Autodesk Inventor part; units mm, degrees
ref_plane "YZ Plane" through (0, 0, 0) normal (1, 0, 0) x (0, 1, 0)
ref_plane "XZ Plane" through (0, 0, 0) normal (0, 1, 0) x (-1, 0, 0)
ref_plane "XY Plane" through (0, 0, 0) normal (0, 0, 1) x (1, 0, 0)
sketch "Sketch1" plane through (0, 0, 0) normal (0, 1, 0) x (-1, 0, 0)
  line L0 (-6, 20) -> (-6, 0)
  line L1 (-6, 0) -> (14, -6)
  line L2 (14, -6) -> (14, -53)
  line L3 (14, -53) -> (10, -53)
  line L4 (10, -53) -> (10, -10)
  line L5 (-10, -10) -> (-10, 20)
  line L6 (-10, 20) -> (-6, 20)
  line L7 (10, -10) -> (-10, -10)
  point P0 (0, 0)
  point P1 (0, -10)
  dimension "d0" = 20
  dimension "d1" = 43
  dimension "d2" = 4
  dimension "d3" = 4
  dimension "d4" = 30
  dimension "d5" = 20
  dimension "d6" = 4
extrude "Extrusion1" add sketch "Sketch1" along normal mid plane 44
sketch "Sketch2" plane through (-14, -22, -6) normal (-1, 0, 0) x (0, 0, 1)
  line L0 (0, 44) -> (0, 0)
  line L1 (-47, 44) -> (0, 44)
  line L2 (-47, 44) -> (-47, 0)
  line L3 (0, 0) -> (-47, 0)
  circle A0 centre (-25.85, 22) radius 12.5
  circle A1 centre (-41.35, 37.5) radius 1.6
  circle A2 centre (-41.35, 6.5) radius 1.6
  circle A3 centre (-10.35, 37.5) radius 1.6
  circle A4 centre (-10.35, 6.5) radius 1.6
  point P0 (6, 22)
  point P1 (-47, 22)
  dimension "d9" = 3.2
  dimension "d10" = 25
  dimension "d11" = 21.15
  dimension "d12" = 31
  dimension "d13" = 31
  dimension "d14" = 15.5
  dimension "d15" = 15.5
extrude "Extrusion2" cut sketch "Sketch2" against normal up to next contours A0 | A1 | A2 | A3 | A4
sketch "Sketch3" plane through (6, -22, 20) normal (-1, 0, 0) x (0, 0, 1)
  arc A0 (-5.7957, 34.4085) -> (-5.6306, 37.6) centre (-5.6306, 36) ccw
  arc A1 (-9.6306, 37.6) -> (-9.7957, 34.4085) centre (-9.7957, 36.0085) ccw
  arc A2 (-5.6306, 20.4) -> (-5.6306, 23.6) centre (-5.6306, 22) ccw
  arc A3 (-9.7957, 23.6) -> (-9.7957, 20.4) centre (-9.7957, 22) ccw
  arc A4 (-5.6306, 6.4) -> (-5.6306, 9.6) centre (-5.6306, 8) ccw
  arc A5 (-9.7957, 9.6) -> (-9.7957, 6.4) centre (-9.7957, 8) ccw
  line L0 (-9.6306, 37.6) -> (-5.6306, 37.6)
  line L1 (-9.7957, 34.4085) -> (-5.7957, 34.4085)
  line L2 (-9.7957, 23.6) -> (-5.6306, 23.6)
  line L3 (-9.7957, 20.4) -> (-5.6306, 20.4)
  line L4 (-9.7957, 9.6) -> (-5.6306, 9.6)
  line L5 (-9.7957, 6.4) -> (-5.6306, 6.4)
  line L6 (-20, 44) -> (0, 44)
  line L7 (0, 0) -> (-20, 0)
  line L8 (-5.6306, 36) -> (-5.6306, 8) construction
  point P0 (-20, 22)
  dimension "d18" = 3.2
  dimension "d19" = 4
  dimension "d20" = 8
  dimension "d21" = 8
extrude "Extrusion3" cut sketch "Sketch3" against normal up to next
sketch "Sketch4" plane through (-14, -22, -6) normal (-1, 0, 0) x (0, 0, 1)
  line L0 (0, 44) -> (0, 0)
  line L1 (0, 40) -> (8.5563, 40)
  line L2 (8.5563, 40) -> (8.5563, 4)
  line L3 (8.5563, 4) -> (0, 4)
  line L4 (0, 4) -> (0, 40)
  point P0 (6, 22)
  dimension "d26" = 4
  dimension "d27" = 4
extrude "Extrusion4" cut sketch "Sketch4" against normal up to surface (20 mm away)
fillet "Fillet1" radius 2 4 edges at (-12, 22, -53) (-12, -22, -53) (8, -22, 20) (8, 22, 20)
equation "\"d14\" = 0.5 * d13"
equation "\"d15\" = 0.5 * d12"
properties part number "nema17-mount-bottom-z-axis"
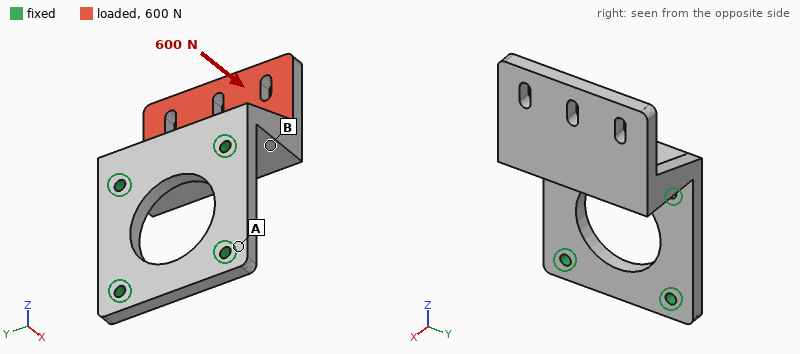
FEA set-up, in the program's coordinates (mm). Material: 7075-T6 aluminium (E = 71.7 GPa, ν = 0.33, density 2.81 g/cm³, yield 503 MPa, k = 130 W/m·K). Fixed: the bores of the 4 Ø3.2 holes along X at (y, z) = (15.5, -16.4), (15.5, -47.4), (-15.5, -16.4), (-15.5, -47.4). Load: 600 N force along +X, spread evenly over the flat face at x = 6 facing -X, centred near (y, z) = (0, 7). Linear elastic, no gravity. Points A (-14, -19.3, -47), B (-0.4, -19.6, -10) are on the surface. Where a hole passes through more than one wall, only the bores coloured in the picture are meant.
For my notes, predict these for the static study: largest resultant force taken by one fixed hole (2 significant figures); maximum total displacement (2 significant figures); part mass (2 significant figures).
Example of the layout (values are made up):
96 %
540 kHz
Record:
350 N
0.49 mm
41 g
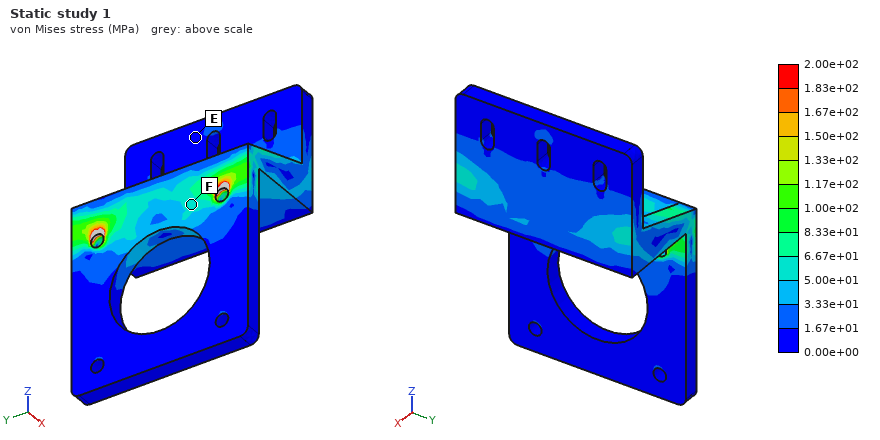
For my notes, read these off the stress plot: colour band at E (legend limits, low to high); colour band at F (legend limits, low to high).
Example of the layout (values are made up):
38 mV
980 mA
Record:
0.00e+00 to 1.67e+01 MPa
5.00e+01 to 6.67e+01 MPa
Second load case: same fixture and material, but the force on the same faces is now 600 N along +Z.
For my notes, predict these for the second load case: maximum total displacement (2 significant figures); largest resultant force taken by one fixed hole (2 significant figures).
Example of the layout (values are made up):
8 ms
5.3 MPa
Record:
0.33 mm
310 N
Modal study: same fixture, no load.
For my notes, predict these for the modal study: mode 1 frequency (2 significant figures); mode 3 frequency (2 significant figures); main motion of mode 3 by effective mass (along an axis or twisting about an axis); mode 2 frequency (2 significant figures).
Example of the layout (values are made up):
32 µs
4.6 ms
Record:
1600 Hz
6000 Hz
along Z
3600 Hz
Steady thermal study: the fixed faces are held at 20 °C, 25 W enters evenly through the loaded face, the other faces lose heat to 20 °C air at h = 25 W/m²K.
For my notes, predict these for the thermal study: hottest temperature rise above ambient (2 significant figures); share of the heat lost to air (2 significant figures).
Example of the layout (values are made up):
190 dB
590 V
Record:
41 K
12 %
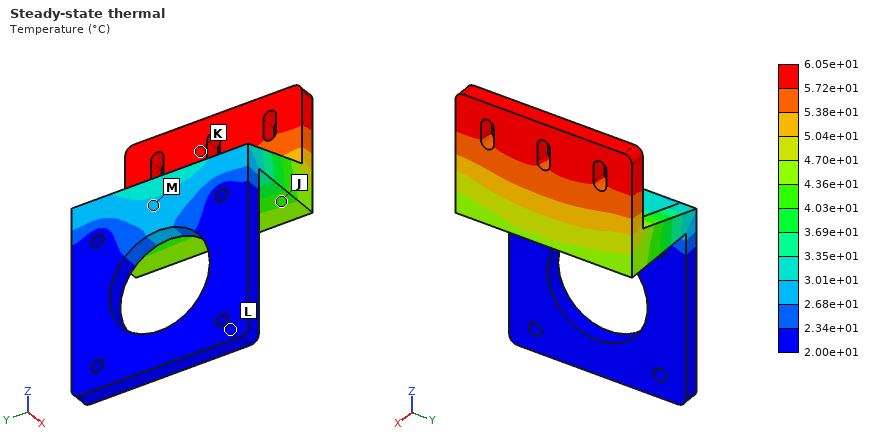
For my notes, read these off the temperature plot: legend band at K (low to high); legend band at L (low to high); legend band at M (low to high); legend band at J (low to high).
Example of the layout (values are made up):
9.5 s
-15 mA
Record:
5.72e+01 to 6.05e+01 °C
2.00e+01 to 2.34e+01 °C
2.68e+01 to 3.01e+01 °C
4.03e+01 to 4.36e+01 °C
